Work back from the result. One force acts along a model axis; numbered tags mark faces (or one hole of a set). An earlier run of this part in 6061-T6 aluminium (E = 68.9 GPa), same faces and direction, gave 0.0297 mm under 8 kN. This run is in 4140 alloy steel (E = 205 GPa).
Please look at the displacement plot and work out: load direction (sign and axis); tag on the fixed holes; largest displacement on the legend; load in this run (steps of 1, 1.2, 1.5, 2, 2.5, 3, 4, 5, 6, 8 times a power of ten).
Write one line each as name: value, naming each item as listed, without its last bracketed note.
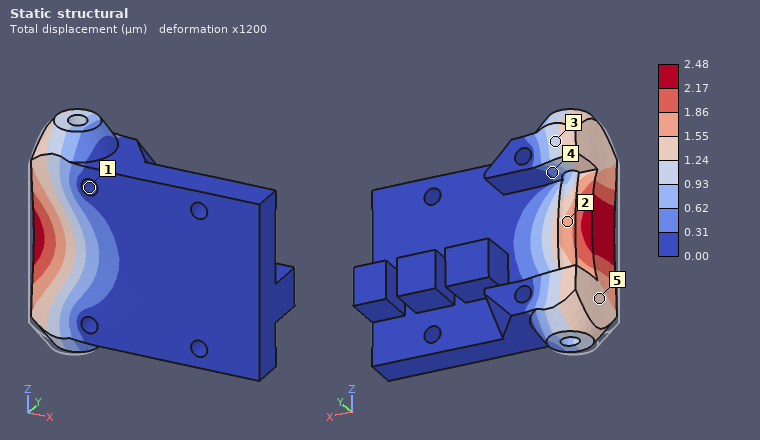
load direction: +Y
tag on the fixed holes: 1
largest displacement on the legend: 2.48 µm
load in this run: 2 kN
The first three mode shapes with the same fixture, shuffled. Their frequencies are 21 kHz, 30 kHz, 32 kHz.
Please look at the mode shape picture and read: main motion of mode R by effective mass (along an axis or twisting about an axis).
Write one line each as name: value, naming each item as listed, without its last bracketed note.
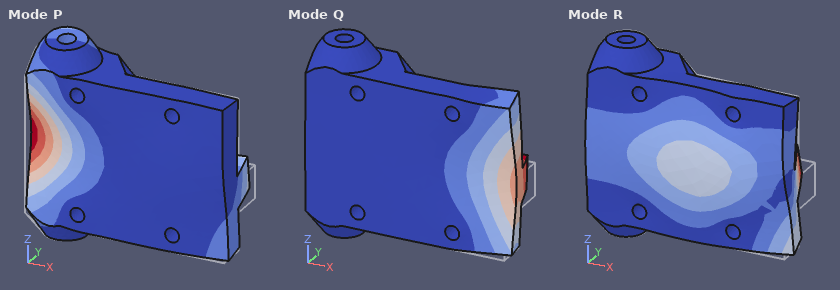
main motion of mode R by effective mass: along Y
